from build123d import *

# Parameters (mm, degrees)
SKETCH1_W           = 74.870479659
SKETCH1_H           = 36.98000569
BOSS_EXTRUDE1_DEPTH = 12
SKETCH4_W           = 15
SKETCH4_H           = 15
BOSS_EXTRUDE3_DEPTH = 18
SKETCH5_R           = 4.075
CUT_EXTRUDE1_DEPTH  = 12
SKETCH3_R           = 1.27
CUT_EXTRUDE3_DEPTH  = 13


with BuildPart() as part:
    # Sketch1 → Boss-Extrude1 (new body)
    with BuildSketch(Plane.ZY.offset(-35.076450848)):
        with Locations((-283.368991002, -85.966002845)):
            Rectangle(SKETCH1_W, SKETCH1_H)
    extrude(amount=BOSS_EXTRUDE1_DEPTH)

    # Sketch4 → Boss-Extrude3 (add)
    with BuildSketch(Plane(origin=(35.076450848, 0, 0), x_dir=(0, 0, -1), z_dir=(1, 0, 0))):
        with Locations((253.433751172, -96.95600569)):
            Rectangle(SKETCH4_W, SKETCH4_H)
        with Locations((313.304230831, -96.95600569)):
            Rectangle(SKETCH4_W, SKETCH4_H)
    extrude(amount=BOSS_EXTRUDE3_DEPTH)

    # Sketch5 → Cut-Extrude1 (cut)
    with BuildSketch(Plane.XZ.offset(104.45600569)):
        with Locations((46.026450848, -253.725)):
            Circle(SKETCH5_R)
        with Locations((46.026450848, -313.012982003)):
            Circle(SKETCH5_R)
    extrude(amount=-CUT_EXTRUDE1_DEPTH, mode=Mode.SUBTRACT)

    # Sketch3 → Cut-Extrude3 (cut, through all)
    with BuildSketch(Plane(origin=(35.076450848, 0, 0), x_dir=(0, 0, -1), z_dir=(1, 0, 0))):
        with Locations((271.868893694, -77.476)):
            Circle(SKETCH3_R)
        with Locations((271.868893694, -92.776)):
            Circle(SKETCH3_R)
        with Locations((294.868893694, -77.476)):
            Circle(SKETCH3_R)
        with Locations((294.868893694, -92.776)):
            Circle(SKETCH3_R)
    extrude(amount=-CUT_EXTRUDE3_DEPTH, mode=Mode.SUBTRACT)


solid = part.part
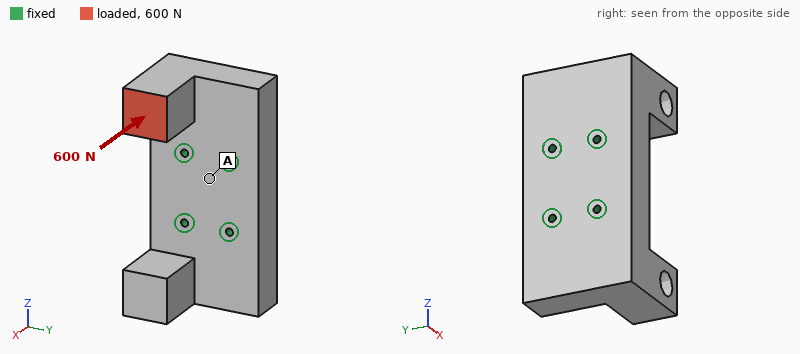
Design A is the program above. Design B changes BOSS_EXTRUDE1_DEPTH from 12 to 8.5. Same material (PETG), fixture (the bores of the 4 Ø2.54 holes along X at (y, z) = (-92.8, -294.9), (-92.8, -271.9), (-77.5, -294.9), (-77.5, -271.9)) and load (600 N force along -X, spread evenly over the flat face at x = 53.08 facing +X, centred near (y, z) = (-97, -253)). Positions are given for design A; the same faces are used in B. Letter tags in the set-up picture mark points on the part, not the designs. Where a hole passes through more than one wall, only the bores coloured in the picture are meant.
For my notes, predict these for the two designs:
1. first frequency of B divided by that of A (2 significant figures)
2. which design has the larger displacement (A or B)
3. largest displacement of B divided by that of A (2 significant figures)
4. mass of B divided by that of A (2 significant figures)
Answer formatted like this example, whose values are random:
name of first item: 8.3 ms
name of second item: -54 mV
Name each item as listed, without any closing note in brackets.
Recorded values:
first frequency of B divided by that of A: 0.71
which design has the larger displacement: B
largest displacement of B divided by that of A: 2.2
mass of B divided by that of A: 0.76
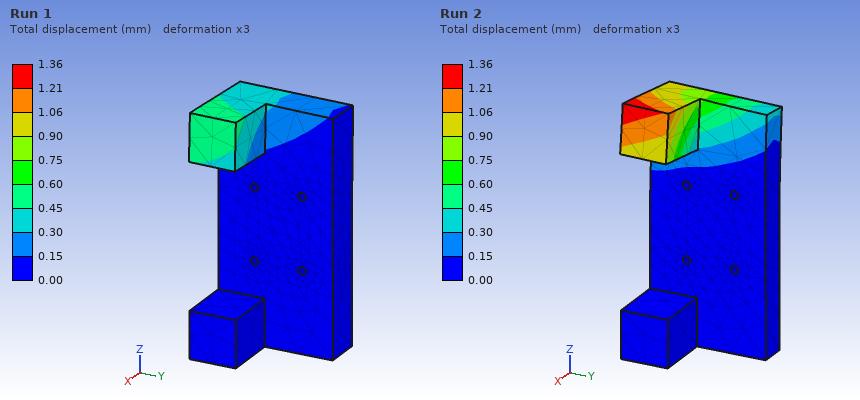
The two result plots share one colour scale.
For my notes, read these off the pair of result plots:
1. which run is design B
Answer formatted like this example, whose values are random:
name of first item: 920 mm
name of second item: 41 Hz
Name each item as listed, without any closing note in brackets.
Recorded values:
which run is design B: Run 2
